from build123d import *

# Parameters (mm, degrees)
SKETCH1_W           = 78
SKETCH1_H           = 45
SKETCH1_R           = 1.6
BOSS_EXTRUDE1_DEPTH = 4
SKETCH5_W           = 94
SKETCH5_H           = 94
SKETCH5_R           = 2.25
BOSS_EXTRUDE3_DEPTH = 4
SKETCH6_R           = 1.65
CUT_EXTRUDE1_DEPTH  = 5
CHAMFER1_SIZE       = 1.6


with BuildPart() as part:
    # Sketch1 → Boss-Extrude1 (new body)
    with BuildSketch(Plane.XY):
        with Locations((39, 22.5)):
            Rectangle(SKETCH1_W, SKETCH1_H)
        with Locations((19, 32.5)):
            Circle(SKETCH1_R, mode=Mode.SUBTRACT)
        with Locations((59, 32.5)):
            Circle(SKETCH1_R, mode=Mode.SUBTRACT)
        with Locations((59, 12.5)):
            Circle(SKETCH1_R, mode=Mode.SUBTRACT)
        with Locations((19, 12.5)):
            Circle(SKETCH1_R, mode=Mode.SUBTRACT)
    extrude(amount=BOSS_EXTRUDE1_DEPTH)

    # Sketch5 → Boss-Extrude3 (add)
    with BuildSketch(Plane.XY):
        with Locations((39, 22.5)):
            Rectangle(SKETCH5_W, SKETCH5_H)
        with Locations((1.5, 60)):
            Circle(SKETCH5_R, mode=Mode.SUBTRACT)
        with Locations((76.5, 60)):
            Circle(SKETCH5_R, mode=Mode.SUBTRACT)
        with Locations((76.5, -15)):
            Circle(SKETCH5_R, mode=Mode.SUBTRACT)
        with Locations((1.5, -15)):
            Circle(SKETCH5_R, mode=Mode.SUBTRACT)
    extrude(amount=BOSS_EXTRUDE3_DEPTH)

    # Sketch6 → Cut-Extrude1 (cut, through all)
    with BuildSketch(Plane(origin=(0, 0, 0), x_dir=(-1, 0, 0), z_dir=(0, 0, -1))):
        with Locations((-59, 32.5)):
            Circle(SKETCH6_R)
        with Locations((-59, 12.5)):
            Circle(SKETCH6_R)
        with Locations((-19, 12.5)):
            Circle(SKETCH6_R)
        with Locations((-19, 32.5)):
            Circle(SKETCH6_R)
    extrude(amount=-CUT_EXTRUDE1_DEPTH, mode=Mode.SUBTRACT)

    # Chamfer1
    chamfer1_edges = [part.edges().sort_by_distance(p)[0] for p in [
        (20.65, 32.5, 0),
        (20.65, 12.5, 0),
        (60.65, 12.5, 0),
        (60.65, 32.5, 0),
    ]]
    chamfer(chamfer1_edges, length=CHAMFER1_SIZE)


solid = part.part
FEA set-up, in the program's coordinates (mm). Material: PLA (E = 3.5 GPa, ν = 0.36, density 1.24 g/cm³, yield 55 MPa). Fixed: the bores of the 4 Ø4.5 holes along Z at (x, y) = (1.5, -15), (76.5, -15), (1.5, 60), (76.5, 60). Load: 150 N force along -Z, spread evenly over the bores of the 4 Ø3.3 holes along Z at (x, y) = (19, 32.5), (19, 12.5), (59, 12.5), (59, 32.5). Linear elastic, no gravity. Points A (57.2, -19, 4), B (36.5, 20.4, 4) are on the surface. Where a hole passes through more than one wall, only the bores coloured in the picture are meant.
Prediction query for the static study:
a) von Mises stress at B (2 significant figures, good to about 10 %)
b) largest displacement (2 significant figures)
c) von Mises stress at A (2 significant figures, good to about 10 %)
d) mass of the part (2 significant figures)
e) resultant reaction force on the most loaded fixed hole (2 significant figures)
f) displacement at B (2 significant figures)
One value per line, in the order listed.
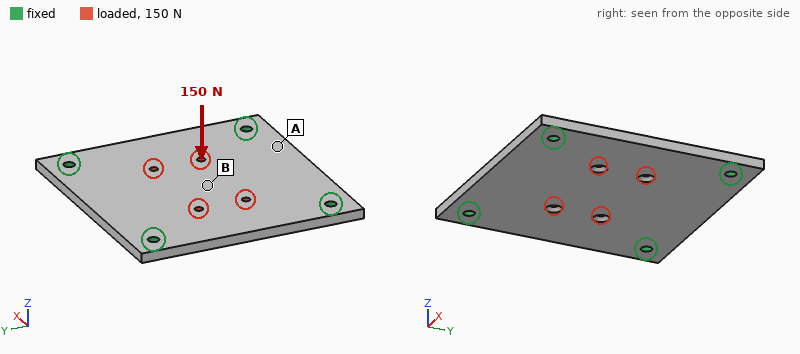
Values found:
4.1 MPa
0.36 mm
1.6 MPa
43 g
38 N
0.36 mm
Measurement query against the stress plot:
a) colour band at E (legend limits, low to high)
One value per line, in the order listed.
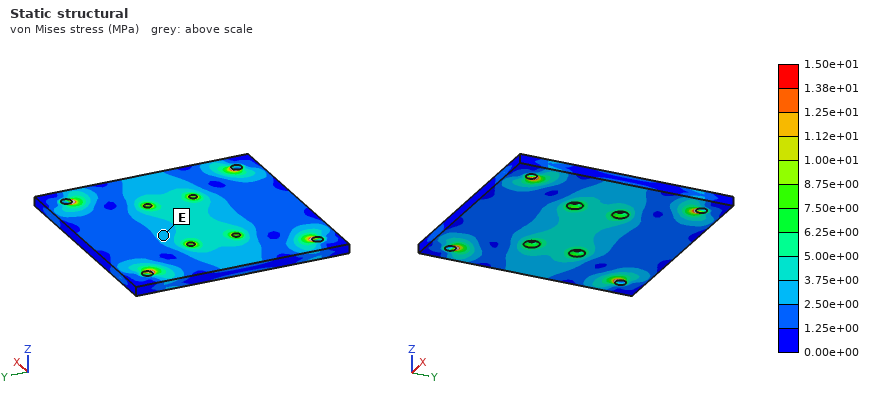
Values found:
2.50e+00 to 3.75e+00 MPa
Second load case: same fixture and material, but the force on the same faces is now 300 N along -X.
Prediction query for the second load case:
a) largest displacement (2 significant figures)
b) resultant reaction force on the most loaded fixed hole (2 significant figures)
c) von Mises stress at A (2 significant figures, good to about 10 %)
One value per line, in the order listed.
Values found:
18 µm
82 N
0.45 MPa
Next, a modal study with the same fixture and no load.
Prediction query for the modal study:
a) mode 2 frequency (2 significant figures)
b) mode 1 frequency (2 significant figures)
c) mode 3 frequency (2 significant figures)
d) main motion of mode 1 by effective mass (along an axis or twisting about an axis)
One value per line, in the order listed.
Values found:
1300 Hz
830 Hz
1300 Hz
along Z
